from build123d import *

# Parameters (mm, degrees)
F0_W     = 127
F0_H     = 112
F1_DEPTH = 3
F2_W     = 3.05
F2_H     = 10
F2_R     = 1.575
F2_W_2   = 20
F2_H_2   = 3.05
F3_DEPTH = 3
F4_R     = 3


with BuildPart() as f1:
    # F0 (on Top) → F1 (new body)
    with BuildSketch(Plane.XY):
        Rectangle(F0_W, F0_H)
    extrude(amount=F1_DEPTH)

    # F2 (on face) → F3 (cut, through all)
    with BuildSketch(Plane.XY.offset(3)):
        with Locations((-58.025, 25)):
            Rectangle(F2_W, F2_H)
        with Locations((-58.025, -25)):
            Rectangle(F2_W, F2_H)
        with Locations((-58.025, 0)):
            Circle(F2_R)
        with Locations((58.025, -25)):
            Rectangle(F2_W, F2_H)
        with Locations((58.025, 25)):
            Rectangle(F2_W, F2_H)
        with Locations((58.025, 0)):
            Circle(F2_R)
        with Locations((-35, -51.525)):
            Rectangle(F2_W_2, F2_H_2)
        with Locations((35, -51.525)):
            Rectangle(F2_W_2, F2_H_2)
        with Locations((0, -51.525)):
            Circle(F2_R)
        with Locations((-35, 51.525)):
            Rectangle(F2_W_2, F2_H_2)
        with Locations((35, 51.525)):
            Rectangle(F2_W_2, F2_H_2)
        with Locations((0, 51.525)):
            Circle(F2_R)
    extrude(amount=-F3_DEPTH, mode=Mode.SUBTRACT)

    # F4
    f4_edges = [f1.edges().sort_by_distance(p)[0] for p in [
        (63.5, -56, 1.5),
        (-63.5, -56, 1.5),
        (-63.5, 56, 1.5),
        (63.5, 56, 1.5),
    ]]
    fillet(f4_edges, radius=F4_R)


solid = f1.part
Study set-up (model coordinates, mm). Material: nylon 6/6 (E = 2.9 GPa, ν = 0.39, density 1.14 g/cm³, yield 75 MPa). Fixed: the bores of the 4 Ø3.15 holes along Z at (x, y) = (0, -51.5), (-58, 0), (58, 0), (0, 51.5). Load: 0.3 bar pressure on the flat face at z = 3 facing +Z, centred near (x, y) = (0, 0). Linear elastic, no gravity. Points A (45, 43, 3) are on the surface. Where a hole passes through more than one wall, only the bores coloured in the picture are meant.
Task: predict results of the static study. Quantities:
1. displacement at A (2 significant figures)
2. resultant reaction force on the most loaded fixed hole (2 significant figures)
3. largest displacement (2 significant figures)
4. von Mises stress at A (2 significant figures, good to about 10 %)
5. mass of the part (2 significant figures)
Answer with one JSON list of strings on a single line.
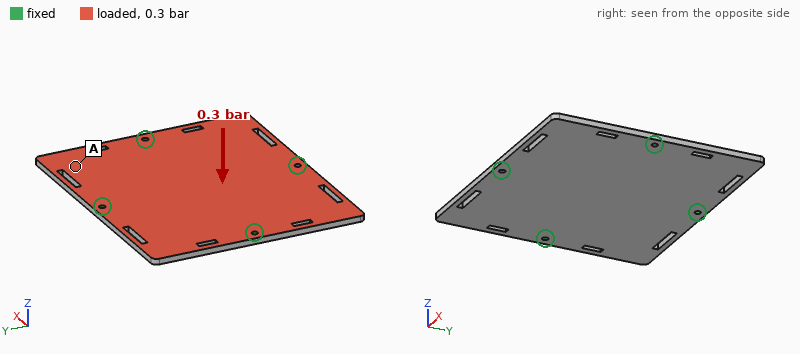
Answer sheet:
["1.1 mm", "100 N", "1.8 mm", "6.1 MPa", "47 g"]
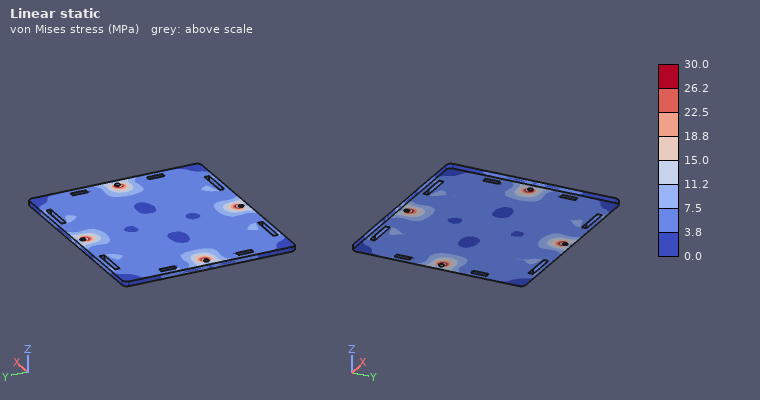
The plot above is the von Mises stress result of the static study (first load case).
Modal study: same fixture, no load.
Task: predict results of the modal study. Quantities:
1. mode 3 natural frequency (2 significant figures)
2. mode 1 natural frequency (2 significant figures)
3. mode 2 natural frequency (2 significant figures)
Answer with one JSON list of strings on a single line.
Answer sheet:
["430 Hz", "390 Hz", "420 Hz"]
